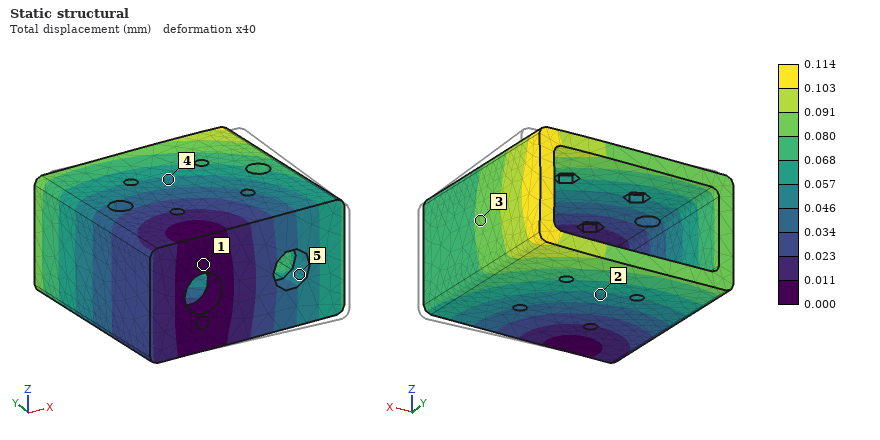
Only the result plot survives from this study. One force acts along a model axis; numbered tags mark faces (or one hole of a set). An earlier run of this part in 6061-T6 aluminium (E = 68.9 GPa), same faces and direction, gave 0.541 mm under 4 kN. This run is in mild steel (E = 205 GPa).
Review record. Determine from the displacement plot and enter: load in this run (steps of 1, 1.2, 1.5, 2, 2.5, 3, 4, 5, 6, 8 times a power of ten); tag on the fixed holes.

2.5 kN
1
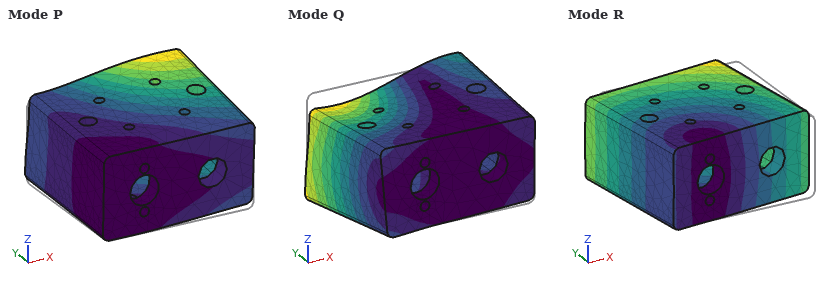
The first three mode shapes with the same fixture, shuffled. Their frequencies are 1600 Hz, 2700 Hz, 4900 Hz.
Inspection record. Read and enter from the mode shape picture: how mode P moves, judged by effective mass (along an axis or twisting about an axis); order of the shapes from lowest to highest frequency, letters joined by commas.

along Z
R, P, Q
